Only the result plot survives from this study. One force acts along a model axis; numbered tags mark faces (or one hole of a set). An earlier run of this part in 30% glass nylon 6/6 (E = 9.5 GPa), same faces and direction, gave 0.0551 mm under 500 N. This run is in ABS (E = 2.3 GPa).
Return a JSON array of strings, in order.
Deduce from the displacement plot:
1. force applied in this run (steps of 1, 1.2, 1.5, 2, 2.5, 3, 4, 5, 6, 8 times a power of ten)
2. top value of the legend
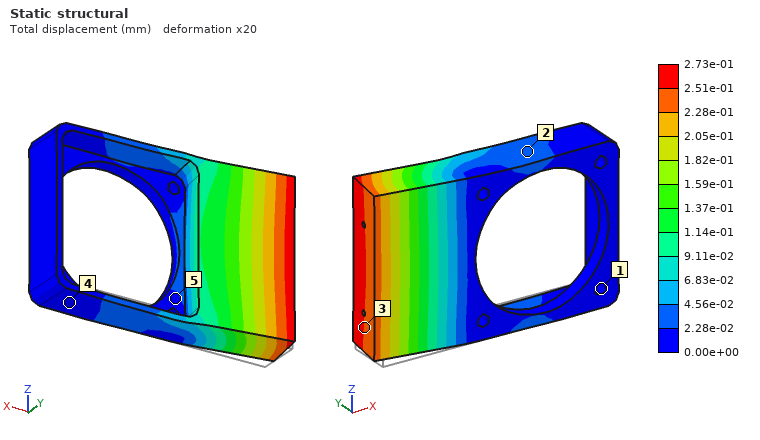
["600 N", "2.73e-01 mm"]
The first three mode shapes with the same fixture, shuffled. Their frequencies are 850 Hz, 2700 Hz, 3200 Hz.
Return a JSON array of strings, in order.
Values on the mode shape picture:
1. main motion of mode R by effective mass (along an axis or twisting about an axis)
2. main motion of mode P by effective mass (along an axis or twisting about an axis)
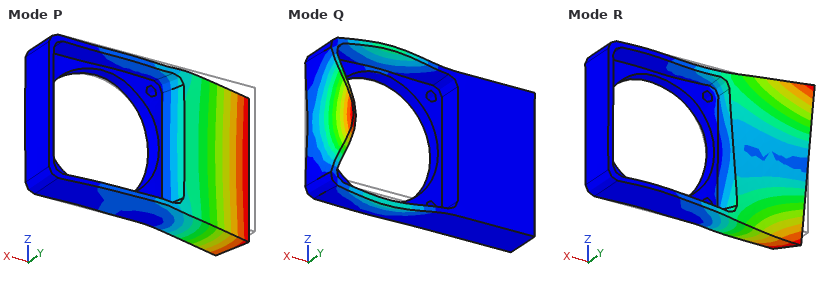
["twisting about X", "along Y"]
